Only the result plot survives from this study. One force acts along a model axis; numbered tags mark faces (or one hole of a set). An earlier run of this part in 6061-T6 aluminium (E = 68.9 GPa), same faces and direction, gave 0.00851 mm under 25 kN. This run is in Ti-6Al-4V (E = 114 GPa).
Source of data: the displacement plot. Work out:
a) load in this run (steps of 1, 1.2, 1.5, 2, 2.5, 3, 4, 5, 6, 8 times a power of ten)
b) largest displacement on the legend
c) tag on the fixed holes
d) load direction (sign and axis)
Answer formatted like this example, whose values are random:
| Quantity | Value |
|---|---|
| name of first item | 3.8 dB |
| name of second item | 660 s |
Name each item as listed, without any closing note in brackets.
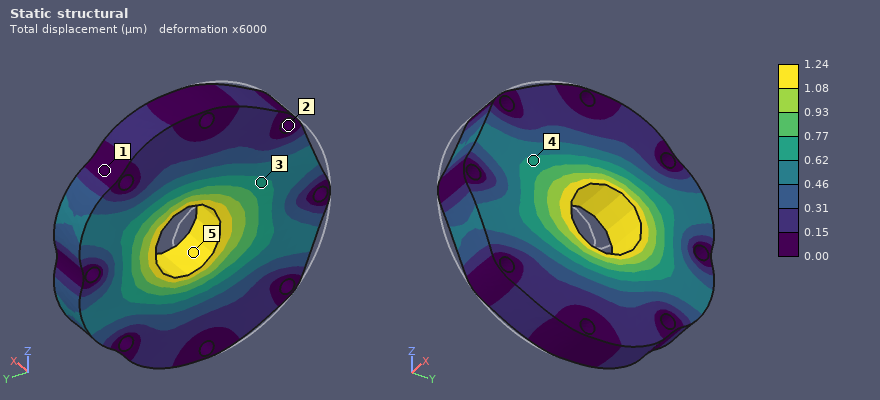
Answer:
| Quantity | Value |
|---|---|
| load in this run | 6 kN |
| largest displacement on the legend | 1.24 µm |
| tag on the fixed holes | 2 |
| load direction | +Y |
